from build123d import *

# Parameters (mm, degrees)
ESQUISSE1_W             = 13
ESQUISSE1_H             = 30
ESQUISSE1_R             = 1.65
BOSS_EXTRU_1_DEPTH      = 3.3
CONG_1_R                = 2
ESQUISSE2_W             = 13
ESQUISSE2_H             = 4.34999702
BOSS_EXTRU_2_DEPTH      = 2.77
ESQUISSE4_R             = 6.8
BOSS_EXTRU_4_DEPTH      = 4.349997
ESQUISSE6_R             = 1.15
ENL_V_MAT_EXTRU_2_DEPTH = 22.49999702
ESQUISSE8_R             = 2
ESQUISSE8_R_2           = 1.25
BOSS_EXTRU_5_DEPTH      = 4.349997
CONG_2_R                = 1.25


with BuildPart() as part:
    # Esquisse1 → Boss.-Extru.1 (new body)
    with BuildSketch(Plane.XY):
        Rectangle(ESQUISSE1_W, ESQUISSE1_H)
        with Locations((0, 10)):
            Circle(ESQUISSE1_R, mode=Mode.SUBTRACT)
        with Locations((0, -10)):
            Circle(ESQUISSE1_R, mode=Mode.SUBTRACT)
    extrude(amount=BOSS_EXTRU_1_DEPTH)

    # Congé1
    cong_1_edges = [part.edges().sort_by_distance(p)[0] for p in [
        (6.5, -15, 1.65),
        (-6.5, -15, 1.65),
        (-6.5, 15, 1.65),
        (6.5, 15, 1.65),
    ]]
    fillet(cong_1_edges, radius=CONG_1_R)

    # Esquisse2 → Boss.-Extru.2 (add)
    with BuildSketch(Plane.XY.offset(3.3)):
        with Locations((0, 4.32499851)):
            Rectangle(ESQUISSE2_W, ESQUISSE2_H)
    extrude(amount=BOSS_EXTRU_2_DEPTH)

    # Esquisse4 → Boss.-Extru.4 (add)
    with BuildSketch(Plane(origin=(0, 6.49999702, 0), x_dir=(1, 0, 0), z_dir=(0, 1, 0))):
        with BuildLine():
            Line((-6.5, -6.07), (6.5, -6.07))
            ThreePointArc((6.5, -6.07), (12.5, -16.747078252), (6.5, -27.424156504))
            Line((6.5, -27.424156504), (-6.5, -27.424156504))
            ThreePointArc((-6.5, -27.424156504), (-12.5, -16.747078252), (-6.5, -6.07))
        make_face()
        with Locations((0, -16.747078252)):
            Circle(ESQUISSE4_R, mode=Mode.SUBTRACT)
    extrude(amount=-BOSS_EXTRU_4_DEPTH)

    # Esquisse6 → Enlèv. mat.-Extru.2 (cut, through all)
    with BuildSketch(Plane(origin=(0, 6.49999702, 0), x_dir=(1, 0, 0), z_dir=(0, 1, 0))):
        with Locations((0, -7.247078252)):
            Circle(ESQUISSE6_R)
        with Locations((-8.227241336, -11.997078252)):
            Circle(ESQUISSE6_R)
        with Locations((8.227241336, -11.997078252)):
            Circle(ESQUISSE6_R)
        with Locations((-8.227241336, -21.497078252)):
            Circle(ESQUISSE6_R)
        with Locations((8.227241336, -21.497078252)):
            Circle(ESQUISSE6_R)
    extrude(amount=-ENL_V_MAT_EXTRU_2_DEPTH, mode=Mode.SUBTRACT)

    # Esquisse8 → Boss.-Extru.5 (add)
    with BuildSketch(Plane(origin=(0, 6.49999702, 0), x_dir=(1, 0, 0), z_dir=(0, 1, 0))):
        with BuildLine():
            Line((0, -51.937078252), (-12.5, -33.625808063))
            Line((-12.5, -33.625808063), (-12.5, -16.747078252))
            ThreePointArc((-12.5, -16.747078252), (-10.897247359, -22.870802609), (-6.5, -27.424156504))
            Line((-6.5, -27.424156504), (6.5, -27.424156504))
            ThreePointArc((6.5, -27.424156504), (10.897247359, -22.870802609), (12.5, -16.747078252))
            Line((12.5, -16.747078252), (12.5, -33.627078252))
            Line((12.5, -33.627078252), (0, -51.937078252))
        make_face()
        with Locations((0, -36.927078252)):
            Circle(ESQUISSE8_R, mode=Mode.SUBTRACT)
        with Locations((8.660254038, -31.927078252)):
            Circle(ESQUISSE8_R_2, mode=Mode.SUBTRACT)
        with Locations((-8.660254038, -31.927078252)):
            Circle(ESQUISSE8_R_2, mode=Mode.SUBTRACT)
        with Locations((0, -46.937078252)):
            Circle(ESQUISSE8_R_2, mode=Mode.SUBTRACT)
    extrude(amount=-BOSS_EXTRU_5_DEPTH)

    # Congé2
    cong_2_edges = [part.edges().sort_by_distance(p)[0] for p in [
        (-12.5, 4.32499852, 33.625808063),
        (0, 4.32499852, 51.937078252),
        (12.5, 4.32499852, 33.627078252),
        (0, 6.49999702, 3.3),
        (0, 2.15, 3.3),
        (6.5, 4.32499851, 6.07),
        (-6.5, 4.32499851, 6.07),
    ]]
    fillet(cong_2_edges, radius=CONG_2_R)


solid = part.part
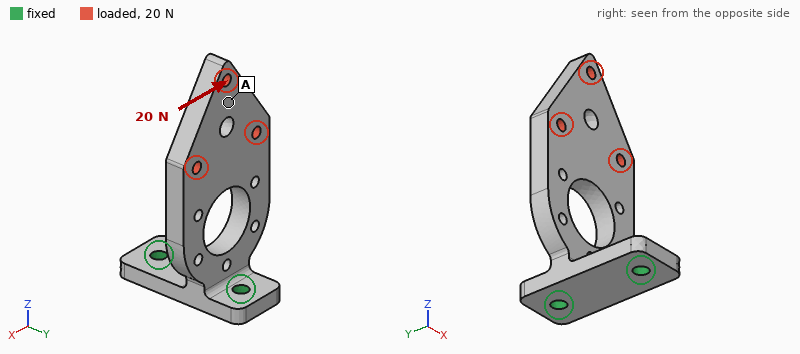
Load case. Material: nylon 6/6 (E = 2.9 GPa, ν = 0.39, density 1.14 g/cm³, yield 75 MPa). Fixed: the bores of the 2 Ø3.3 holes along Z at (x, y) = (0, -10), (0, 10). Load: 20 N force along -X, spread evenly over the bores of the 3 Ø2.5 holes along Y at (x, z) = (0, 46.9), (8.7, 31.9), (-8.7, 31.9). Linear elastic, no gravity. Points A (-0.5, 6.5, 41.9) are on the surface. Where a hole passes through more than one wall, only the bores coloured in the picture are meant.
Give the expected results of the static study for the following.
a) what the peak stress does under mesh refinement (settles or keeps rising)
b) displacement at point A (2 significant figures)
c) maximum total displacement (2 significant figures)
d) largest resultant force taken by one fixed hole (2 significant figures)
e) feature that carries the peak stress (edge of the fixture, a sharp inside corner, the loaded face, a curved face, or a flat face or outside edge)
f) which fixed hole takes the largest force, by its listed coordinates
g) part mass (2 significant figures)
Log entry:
keeps rising
0.61 mm
0.75 mm
18 N
edge of the fixture
(0, 10)
5.0 g
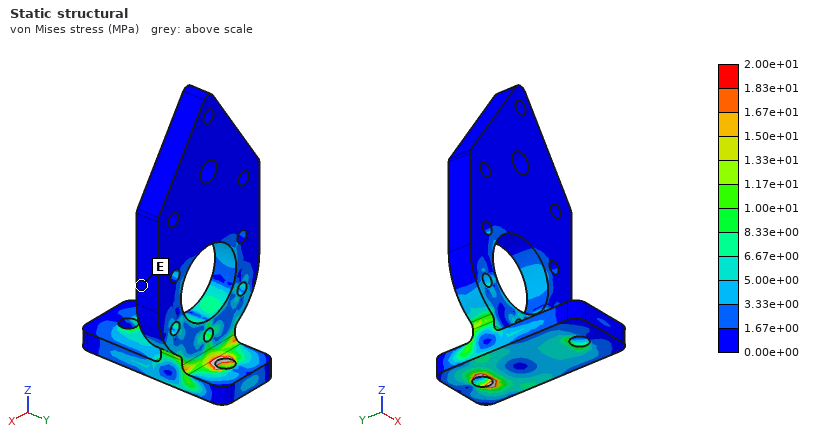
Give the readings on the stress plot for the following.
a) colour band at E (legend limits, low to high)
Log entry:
0.00e+00 to 1.67e+00 MPa
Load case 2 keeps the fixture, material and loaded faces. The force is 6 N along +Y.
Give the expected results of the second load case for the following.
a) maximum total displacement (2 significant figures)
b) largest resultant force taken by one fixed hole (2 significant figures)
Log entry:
0.76 mm
13 N
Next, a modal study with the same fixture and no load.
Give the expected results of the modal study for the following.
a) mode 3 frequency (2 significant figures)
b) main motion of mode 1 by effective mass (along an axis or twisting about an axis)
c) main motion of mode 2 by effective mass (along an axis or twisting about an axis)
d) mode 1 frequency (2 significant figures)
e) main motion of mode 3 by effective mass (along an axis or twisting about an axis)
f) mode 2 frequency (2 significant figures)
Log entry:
1600 Hz
along Y
along X
400 Hz
twisting about Z
650 Hz
